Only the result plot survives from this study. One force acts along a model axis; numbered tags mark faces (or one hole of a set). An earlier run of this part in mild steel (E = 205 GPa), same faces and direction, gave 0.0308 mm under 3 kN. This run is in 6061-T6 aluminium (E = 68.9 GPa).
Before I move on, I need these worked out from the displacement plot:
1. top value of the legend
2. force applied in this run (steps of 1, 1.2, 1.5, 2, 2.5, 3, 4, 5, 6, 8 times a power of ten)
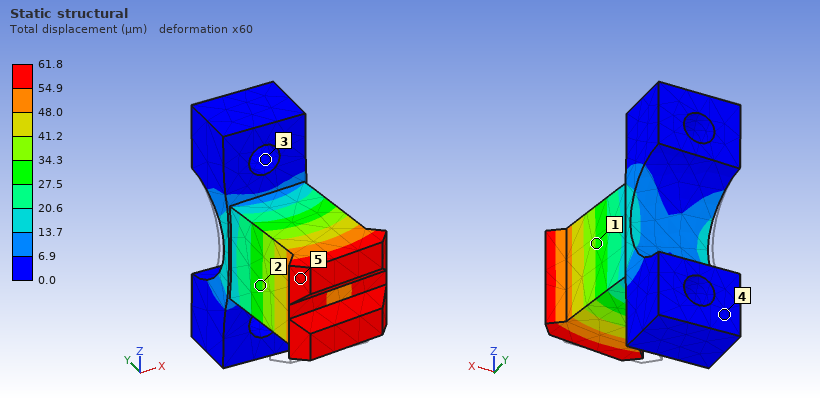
61.8 µm
2 kN
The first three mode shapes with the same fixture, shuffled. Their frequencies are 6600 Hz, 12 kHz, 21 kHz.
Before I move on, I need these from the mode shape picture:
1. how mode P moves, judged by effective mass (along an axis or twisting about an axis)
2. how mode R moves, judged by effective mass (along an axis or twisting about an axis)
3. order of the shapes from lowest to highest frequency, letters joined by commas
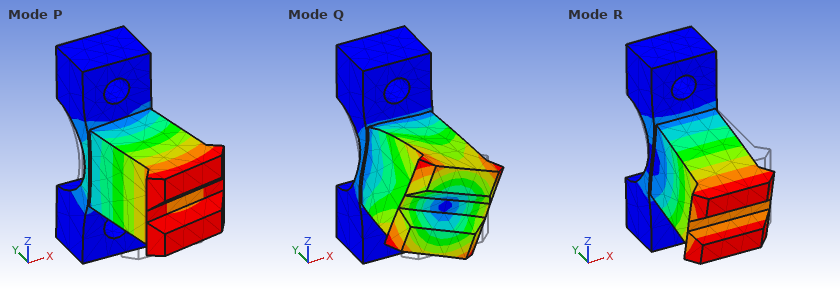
along X
along Z
P, R, Q
